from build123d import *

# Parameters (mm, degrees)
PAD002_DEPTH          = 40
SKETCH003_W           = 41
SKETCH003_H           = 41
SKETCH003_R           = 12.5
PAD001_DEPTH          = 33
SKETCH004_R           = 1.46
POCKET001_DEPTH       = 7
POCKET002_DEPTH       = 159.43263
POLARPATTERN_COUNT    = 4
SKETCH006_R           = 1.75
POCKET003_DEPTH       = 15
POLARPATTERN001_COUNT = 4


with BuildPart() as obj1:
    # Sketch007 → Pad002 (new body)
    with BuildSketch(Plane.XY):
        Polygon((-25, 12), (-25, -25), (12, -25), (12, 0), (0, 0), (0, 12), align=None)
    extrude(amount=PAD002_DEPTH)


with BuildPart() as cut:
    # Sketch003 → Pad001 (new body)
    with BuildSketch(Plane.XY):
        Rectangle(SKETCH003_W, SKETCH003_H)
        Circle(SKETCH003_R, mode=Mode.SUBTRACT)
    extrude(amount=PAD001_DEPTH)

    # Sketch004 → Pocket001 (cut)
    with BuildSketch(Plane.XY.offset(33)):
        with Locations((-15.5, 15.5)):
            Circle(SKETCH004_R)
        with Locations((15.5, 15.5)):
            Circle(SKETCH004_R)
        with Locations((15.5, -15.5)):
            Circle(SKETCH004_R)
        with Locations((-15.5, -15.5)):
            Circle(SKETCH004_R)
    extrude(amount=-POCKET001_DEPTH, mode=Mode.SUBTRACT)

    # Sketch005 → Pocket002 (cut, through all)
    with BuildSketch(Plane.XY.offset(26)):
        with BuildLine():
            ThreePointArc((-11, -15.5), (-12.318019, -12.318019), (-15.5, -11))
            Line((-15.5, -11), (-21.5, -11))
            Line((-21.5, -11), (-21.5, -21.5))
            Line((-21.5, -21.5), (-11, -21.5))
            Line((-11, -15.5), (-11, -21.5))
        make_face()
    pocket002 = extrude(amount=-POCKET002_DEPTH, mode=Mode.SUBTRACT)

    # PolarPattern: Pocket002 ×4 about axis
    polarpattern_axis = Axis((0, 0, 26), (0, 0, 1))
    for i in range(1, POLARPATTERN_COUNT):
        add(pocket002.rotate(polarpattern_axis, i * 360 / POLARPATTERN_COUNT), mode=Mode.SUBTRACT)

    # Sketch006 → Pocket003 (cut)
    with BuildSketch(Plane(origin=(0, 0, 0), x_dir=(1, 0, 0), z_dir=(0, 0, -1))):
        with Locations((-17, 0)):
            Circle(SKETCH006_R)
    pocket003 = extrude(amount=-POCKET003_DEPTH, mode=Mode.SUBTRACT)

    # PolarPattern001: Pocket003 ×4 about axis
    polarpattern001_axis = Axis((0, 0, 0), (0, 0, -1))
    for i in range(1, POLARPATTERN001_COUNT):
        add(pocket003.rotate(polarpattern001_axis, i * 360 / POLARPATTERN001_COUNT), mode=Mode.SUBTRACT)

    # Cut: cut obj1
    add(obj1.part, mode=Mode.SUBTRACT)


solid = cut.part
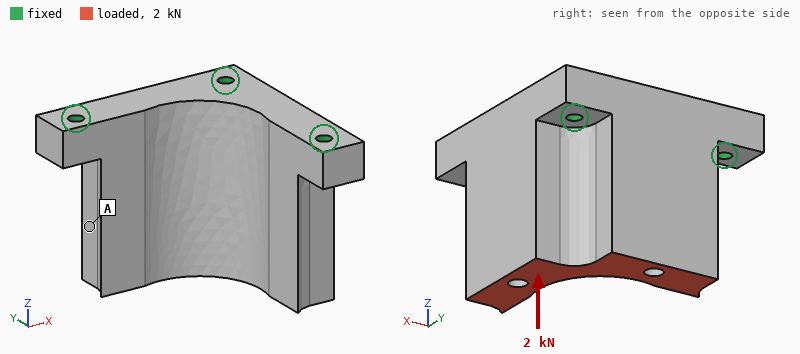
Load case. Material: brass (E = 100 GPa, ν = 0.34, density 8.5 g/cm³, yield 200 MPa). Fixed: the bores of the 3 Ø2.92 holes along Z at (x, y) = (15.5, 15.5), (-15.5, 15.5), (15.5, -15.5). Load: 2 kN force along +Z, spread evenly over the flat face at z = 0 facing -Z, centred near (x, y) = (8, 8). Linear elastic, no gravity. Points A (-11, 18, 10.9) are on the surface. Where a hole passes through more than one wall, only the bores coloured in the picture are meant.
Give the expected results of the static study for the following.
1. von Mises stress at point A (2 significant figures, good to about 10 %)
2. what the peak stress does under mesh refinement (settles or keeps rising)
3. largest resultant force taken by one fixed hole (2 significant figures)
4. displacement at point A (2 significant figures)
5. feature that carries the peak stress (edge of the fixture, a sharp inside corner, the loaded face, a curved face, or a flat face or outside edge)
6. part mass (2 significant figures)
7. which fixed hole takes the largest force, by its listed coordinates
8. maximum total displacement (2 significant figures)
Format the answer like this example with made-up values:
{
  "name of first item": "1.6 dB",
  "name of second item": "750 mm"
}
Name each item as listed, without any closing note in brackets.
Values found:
{
  "von Mises stress at point A": "5.0 MPa",
  "what the peak stress does under mesh refinement": "keeps rising",
  "largest resultant force taken by one fixed hole": "1.1 kN",
  "displacement at point A": "3.1 µm",
  "feature that carries the peak stress": "edge of the fixture",
  "part mass": "120 g",
  "which fixed hole takes the largest force, by its listed coordinates": "(15.5, 15.5)",
  "maximum total displacement": "3.9 µm"
}
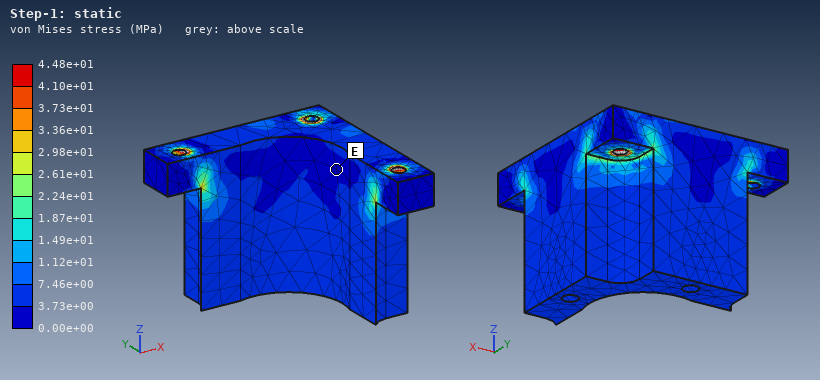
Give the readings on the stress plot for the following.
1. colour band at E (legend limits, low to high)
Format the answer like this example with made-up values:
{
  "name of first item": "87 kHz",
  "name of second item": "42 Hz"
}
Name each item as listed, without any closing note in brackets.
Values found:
{
  "colour band at E": "0.00e+00 to 3.73e+00 MPa"
}
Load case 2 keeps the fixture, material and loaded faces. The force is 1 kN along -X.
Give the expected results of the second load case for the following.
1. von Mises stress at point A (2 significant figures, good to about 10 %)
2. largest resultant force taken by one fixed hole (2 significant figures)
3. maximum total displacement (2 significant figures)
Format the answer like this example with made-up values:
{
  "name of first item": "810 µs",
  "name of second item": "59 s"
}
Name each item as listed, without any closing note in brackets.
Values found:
{
  "von Mises stress at point A": "7.7 MPa",
  "largest resultant force taken by one fixed hole": "1.1 kN",
  "maximum total displacement": "31 µm"
}
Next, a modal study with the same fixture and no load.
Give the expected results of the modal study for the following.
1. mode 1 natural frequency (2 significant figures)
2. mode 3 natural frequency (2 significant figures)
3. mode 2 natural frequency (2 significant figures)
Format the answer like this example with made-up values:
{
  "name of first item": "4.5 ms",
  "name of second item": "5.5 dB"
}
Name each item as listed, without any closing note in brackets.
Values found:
{
  "mode 1 natural frequency": "5500 Hz",
  "mode 3 natural frequency": "10 kHz",
  "mode 2 natural frequency": "6300 Hz"
}
